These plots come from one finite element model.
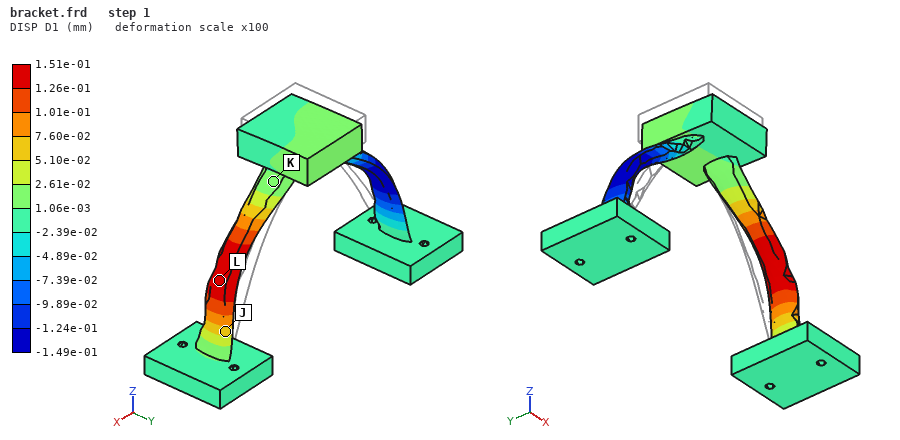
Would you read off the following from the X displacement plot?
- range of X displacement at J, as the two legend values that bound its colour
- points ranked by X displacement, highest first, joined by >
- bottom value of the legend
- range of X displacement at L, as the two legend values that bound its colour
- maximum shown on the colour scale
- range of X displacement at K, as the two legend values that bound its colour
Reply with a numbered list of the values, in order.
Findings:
1. 5.10e-02 to 7.60e-02 mm
2. L > J > K
3. -1.49e-01 mm
4. 1.26e-01 to 1.51e-01 mm
5. 1.51e-01 mm
6. 1.06e-03 to 2.61e-02 mm
